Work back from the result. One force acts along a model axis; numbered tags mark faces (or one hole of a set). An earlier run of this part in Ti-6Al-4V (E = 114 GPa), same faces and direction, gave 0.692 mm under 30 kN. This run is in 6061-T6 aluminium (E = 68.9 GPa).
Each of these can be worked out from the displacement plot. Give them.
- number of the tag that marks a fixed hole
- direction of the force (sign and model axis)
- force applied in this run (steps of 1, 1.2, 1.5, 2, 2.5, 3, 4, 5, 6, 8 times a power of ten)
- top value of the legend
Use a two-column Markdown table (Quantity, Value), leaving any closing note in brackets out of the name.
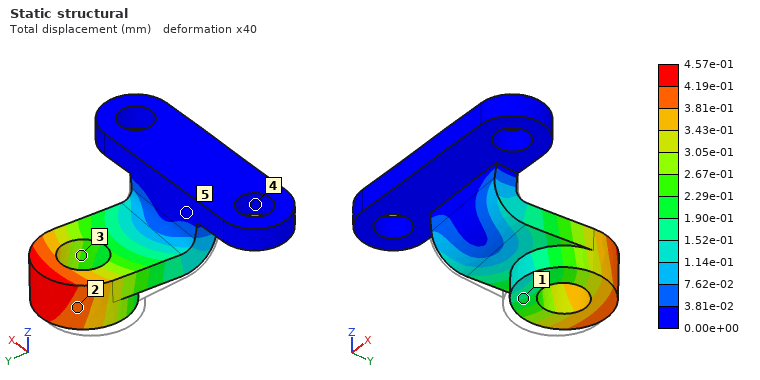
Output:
| Quantity | Value |
|---|---|
| number of the tag that marks a fixed hole | 4 |
| direction of the force | +X |
| force applied in this run | 12 kN |
| top value of the legend | 4.57e-01 mm |
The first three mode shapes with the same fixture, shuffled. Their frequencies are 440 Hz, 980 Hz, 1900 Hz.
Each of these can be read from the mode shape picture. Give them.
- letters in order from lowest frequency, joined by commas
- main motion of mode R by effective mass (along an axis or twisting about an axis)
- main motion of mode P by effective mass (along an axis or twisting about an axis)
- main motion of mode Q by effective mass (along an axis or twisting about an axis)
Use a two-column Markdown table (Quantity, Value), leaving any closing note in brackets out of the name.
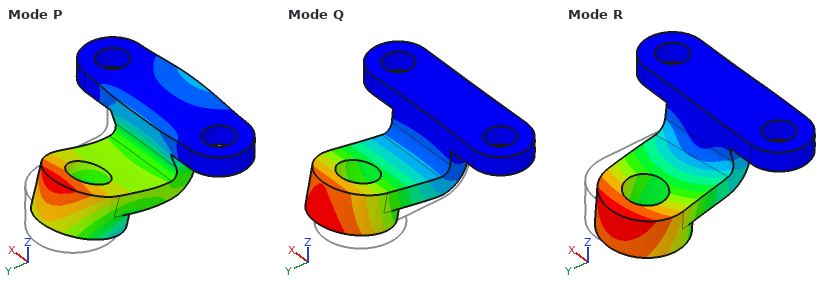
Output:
| Quantity | Value |
|---|---|
| letters in order from lowest frequency, joined by commas | Q, R, P |
| main motion of mode R by effective mass | along X |
| main motion of mode P by effective mass | along Y |
| main motion of mode Q by effective mass | along Z |
